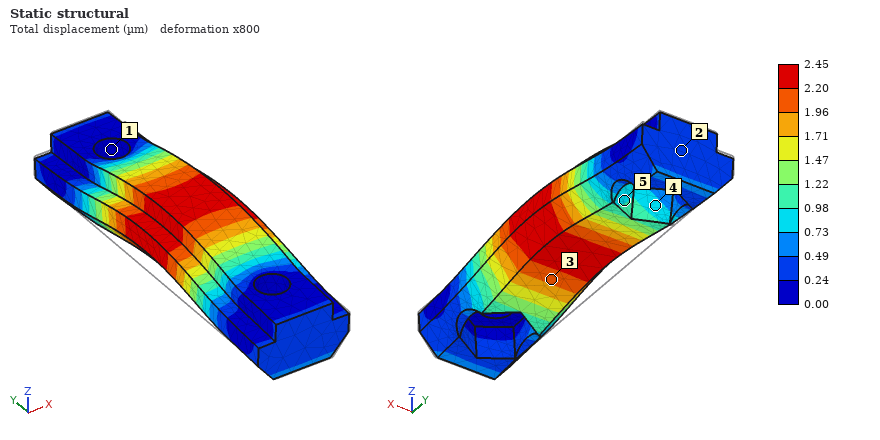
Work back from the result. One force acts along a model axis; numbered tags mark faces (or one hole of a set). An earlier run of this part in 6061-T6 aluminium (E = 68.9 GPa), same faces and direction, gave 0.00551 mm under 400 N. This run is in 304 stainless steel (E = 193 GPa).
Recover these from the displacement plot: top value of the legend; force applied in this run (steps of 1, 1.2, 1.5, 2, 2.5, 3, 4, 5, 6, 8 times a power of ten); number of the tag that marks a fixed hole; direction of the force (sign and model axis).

2.45 µm
500 N
1
+Z
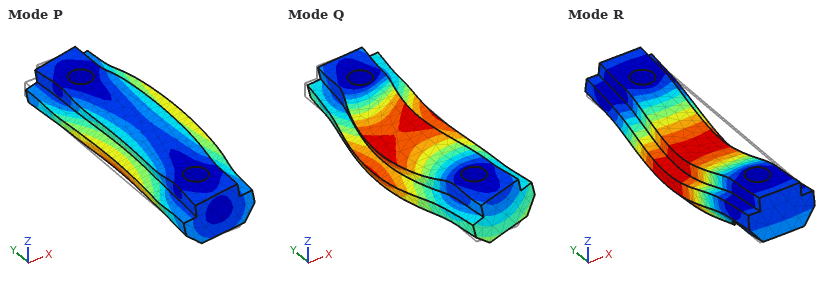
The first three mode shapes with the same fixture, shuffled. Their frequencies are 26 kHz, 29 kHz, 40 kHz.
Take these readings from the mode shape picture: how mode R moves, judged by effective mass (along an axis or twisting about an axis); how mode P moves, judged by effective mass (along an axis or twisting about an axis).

along Z
along X
